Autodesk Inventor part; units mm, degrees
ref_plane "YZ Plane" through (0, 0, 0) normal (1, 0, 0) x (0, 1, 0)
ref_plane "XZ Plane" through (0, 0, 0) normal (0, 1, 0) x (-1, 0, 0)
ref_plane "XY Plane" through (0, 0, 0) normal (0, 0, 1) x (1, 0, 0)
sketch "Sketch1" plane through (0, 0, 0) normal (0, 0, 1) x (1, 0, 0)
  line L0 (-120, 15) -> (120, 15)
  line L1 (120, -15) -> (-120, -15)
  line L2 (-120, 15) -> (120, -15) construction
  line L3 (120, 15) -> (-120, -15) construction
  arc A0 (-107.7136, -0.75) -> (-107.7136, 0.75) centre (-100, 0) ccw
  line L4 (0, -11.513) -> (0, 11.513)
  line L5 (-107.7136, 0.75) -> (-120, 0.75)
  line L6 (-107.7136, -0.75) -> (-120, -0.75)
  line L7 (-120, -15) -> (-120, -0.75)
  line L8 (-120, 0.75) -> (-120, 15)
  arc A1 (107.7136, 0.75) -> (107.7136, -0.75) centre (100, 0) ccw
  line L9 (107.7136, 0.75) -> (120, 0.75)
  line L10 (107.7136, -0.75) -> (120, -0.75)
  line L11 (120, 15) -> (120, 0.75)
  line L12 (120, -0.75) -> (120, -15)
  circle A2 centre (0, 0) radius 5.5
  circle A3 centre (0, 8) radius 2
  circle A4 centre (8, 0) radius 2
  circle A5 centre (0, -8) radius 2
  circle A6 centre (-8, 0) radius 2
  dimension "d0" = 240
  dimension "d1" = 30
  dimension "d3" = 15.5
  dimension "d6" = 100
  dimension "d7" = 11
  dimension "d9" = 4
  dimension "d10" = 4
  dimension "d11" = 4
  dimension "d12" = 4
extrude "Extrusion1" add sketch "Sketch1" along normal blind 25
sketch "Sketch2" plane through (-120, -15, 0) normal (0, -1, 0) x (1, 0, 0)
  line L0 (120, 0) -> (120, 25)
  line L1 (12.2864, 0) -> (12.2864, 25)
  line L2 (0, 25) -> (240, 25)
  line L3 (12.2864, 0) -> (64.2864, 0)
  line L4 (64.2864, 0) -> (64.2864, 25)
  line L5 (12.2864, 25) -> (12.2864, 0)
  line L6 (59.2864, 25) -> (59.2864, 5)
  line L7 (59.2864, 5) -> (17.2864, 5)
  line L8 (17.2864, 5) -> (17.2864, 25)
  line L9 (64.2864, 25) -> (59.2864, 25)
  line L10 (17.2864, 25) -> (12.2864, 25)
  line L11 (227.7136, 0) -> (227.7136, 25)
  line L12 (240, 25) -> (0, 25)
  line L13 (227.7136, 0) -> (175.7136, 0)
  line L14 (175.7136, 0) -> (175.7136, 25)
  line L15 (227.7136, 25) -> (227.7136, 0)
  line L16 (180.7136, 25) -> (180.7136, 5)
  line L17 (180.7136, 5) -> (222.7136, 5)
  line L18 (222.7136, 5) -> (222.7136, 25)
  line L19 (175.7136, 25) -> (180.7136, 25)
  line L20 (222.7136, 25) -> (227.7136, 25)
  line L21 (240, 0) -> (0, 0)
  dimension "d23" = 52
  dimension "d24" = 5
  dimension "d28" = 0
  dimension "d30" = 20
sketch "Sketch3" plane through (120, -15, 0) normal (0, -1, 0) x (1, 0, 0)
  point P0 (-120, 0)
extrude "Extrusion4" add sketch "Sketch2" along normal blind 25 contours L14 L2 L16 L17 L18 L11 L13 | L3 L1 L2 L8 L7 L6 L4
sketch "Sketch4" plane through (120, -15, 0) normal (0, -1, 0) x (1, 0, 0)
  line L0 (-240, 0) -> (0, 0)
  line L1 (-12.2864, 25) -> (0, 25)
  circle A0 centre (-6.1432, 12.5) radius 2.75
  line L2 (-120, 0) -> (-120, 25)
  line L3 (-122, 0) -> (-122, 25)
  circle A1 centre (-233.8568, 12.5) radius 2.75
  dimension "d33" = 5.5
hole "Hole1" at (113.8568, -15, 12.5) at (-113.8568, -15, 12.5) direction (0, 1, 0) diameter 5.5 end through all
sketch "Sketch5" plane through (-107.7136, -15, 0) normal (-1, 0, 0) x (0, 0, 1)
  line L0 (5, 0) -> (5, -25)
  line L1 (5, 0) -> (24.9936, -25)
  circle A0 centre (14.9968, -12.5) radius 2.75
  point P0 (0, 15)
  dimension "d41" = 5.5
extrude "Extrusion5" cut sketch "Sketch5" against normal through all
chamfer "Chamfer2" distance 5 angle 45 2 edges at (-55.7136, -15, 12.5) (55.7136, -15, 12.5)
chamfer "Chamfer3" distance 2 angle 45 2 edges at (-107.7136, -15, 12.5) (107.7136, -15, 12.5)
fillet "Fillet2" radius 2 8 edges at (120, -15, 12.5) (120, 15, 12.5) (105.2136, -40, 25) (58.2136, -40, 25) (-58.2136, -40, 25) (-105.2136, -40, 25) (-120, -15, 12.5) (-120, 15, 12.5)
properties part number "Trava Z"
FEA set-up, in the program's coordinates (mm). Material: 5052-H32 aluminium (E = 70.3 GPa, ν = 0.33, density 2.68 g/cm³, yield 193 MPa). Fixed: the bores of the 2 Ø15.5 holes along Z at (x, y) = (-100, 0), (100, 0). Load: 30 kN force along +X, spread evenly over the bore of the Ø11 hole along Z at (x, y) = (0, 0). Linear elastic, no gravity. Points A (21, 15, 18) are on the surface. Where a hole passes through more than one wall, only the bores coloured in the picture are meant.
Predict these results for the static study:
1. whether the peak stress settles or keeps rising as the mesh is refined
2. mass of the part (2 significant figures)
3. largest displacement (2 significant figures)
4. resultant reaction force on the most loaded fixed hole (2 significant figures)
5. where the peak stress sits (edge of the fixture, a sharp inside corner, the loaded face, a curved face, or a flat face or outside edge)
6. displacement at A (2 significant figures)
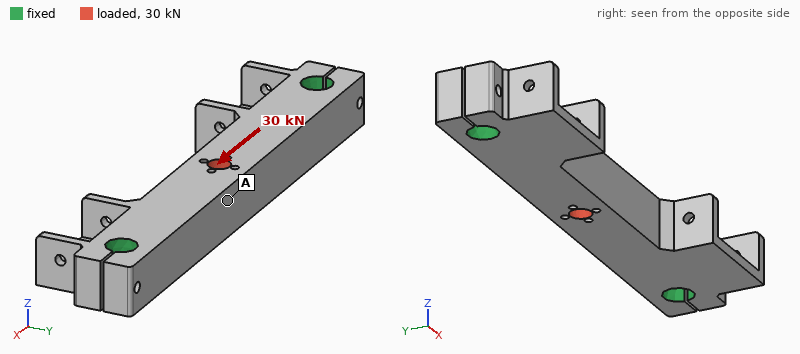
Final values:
keeps rising
500 g
36 µm
15 kN
a sharp inside corner
21 µm
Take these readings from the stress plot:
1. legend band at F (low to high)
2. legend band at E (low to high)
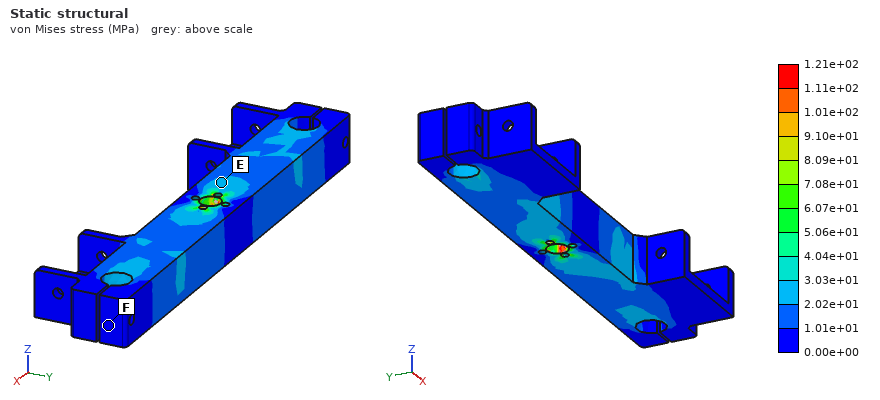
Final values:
0.00e+00 to 1.01e+01 MPa
2.02e+01 to 3.03e+01 MPa
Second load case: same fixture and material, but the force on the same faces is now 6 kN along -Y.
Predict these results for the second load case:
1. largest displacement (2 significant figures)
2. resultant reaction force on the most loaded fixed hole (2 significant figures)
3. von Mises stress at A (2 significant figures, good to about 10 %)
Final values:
81 µm
3.0 kN
21 MPa
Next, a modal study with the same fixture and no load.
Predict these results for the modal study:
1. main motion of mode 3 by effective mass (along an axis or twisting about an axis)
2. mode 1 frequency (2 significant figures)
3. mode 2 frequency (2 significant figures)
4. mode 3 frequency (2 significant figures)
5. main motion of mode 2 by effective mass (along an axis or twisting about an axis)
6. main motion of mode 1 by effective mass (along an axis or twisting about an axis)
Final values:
twisting about X
3200 Hz
3600 Hz
6400 Hz
along Y
along Z
